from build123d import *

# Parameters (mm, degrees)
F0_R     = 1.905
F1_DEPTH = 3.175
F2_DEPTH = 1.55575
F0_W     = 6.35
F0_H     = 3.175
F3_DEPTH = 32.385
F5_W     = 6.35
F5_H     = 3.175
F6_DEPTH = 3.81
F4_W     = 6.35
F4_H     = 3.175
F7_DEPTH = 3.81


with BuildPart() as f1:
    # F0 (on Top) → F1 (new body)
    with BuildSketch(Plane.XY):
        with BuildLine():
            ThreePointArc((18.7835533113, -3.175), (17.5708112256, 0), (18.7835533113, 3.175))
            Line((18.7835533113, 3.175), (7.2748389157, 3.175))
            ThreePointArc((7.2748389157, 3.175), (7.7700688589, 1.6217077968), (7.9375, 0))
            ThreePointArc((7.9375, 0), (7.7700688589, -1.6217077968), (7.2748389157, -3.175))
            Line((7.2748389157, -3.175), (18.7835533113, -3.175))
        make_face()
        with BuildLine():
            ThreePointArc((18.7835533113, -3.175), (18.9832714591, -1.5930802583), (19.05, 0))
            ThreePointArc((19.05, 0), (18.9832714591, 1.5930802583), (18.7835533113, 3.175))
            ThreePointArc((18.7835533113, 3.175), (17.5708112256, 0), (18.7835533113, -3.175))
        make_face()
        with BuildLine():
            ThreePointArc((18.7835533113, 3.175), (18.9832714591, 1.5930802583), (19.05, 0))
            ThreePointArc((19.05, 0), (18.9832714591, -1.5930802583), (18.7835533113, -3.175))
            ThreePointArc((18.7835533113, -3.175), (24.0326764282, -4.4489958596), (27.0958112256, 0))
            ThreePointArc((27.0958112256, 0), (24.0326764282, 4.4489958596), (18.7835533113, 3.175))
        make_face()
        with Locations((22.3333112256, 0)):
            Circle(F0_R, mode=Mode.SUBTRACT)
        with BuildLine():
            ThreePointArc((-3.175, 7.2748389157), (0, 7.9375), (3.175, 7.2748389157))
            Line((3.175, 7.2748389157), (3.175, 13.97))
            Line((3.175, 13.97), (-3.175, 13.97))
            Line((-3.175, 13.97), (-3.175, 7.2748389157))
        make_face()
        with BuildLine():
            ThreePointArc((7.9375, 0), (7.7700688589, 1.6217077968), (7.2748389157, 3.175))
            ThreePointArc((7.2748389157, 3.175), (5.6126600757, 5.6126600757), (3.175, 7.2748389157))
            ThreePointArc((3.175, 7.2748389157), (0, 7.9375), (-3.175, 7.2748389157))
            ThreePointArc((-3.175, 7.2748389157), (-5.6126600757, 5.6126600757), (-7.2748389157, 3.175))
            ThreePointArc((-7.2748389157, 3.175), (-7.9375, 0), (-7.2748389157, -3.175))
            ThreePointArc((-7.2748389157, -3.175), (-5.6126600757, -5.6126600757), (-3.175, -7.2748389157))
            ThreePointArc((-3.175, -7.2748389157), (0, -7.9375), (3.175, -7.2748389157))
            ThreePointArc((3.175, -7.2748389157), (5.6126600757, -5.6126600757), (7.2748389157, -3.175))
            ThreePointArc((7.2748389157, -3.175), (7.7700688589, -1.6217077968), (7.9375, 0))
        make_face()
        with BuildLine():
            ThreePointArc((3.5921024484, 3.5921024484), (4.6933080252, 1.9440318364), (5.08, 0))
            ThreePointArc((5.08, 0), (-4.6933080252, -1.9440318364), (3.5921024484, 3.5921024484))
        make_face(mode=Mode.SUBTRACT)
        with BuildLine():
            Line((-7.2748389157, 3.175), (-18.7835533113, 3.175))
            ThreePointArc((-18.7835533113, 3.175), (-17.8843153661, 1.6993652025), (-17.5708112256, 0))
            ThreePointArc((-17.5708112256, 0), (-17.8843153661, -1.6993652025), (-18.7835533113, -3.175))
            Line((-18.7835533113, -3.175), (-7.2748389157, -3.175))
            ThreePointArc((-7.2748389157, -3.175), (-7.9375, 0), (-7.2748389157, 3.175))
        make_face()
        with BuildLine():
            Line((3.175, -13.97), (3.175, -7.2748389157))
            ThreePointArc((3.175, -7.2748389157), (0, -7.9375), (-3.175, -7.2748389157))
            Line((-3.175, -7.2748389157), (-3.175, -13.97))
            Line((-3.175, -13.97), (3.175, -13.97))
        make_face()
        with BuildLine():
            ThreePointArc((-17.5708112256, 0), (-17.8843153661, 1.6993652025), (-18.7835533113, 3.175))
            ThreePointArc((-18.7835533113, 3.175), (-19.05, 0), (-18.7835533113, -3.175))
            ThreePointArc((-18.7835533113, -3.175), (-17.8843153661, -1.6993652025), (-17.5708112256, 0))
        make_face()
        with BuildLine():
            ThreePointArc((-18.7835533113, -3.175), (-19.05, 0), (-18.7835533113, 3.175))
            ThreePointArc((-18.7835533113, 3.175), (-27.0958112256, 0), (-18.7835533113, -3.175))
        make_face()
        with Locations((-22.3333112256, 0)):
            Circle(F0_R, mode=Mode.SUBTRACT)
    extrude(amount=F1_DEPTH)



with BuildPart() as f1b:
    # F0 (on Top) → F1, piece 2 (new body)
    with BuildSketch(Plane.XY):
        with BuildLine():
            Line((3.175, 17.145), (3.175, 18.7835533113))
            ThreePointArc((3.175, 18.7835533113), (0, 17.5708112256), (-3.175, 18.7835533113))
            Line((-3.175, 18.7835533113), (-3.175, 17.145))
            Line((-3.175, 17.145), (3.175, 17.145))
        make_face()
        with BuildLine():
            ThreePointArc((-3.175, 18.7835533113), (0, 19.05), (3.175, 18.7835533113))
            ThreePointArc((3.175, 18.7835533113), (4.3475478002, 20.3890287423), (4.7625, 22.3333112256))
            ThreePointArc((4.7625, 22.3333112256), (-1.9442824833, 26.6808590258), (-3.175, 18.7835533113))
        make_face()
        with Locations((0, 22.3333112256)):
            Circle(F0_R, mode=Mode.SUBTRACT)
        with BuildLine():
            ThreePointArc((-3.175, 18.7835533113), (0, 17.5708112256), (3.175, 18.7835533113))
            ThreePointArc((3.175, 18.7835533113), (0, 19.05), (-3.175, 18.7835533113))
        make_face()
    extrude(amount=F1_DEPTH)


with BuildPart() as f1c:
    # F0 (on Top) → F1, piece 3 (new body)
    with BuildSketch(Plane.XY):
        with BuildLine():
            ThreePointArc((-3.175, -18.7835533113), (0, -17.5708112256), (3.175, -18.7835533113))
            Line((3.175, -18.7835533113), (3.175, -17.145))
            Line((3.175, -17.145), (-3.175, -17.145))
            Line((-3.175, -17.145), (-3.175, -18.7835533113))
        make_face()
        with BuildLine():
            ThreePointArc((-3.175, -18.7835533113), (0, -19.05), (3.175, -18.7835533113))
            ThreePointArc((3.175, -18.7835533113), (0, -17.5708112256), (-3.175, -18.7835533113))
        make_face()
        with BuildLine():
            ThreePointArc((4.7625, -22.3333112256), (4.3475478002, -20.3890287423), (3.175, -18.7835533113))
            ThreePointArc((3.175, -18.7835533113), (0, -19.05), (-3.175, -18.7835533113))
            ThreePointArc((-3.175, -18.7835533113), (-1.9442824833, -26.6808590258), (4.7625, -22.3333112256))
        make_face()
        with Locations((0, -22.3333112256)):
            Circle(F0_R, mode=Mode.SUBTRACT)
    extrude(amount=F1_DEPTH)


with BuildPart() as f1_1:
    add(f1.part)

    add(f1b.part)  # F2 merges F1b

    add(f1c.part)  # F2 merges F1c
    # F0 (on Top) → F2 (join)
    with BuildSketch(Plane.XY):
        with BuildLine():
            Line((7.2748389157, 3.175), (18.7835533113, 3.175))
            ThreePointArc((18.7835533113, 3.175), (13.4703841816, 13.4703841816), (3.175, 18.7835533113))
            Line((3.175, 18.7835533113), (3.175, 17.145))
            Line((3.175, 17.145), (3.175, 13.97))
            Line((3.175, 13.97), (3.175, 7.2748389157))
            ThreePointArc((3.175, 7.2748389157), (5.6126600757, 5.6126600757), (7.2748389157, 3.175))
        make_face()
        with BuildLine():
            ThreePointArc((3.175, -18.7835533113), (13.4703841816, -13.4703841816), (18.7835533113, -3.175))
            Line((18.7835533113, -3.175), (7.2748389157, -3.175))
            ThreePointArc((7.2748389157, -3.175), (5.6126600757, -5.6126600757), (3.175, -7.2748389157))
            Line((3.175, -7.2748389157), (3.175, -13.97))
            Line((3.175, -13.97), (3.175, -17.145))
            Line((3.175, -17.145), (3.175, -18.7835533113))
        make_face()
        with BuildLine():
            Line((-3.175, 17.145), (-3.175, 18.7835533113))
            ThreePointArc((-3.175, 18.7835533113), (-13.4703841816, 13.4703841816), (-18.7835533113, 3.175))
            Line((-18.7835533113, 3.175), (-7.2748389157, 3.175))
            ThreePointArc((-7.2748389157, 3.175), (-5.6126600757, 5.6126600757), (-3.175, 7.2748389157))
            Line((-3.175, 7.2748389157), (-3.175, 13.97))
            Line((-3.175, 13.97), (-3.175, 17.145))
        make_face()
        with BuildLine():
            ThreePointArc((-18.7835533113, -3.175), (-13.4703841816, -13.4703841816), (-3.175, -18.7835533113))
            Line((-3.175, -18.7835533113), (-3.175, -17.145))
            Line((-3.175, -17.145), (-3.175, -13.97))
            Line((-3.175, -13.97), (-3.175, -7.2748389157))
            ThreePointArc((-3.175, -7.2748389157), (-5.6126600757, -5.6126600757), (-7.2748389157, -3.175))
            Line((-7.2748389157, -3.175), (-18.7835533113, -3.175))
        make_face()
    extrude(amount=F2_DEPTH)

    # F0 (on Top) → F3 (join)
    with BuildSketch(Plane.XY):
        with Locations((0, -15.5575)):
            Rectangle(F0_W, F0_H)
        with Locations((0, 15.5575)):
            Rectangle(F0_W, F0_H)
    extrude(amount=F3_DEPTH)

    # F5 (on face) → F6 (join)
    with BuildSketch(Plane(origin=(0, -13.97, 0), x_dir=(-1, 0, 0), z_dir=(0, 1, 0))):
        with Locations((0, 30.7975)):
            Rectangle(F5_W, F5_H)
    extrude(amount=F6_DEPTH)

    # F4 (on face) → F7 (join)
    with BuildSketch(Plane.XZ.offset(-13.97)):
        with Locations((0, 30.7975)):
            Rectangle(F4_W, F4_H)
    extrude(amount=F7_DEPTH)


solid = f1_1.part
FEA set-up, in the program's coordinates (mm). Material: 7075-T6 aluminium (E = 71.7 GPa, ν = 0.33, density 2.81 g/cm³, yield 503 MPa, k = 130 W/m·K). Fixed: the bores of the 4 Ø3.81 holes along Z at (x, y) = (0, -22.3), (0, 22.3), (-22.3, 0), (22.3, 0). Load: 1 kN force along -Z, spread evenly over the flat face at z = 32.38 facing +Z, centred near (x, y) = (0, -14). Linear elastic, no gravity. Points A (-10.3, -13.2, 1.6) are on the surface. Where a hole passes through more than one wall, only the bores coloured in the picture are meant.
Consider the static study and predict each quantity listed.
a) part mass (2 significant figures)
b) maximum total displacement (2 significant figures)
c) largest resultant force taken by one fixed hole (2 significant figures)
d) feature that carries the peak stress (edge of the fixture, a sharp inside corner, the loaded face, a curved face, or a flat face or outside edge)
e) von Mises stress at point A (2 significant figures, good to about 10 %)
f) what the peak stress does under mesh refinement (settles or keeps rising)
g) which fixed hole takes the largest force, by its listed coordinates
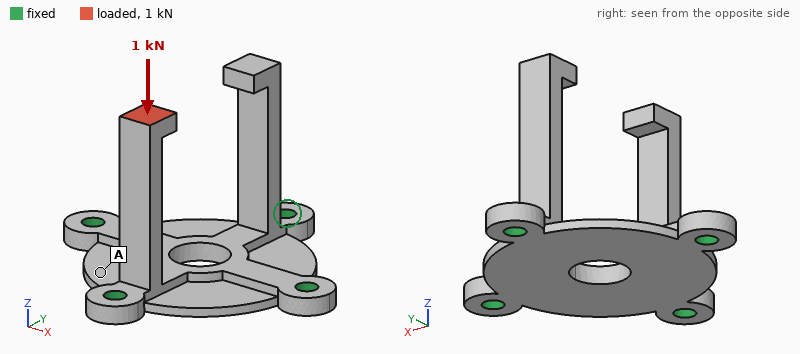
12 g
0.97 mm
830 N
edge of the fixture
37 MPa
keeps rising
(0, -22.3)
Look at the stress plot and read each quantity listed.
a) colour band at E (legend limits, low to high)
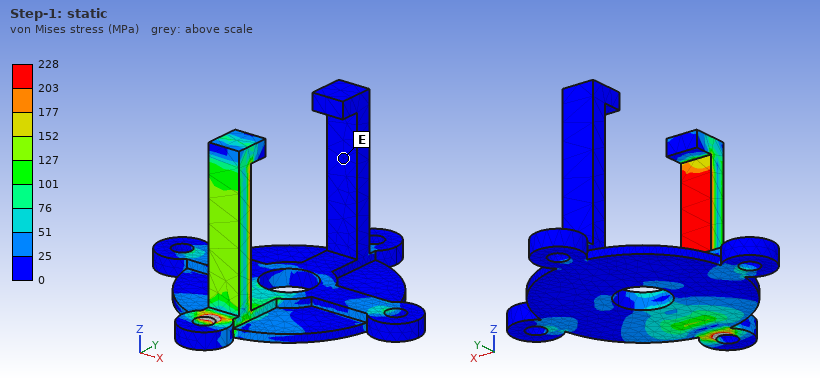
0 to 25 MPa
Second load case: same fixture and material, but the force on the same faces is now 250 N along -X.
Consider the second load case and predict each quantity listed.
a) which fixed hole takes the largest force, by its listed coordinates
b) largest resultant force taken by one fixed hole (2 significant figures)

(0, -22.3)
360 N
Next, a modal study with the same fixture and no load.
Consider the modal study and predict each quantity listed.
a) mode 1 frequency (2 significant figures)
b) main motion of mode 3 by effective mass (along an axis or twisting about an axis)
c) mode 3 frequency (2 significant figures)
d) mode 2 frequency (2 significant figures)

2100 Hz
along X
3300 Hz
2200 Hz
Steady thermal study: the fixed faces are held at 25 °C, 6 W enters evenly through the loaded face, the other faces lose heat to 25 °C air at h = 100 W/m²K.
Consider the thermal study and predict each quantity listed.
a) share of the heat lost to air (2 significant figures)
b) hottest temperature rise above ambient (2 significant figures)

38 %
57 K
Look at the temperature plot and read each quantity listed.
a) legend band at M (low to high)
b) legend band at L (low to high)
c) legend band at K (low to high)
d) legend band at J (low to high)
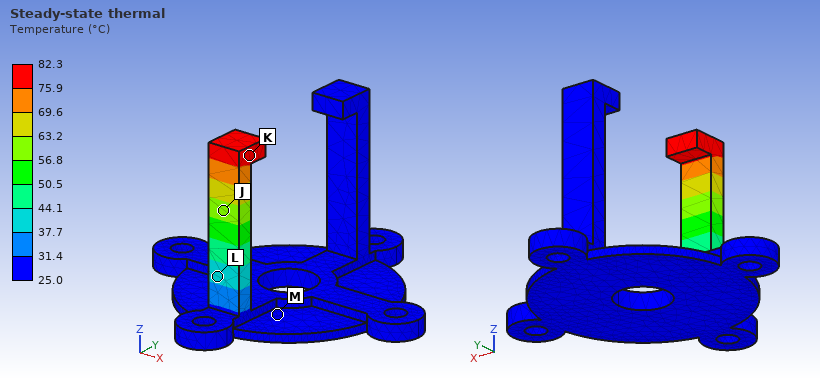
25.0 to 31.4 °C
37.7 to 44.1 °C
75.9 to 82.3 °C
56.8 to 63.2 °C
